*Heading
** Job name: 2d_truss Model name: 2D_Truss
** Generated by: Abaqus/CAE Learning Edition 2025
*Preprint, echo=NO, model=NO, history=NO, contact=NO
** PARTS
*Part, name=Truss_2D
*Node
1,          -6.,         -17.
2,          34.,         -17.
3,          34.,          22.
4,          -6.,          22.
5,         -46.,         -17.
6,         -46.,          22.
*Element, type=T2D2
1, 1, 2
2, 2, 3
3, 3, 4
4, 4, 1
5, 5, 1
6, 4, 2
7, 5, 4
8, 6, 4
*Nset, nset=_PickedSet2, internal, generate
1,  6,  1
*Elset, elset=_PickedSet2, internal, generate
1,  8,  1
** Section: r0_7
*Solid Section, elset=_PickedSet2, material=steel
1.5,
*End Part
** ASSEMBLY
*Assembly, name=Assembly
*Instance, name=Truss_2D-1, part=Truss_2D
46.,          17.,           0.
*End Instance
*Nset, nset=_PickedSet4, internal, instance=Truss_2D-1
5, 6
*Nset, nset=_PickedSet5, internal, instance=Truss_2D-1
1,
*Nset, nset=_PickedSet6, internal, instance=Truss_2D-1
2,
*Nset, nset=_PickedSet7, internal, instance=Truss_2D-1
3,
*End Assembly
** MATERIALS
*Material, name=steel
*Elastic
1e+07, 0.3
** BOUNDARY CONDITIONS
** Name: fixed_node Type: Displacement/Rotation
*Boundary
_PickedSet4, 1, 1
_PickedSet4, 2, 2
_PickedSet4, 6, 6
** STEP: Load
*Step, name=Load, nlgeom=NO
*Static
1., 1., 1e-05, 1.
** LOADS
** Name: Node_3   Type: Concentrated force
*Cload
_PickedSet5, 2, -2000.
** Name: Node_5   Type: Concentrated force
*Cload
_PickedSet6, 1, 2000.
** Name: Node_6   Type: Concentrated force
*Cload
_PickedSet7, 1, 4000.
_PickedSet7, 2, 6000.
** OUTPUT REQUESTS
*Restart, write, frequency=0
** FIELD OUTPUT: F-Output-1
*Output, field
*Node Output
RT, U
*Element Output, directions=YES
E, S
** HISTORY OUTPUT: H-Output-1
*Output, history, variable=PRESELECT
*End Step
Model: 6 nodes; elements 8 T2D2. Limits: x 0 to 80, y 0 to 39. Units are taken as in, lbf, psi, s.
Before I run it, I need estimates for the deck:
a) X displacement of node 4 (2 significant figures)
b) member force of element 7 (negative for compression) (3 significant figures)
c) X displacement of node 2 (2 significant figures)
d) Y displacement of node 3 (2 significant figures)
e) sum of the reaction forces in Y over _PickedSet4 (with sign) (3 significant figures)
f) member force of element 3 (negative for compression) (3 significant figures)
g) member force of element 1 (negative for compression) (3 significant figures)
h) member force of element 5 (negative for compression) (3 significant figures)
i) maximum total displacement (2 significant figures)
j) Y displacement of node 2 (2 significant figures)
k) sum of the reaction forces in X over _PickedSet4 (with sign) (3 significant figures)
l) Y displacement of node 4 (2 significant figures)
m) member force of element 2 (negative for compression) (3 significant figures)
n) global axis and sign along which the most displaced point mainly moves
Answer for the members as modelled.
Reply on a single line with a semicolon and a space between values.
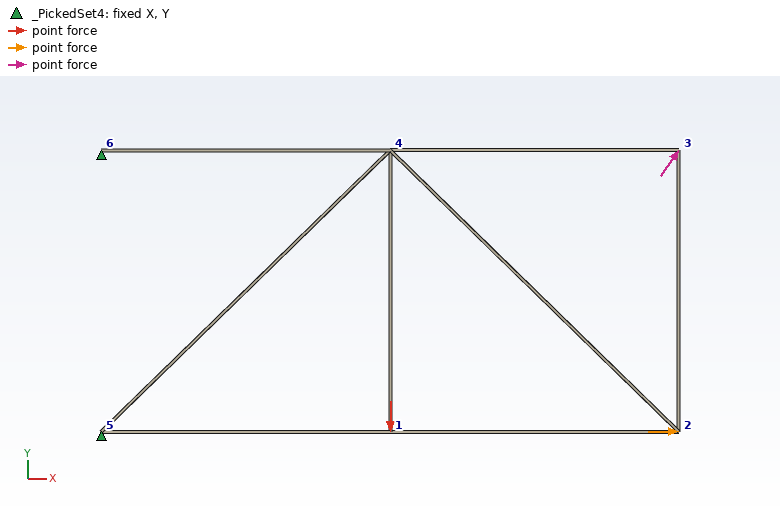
-0.017 in; 5730 lbf; 0.043 in; 0.17 in; -4000 lbf; 4000 lbf; 8150 lbf; 8150 lbf; 0.17 in; 0.16 in; -6000 lbf; 0.048 in; 6000 lbf; +Y
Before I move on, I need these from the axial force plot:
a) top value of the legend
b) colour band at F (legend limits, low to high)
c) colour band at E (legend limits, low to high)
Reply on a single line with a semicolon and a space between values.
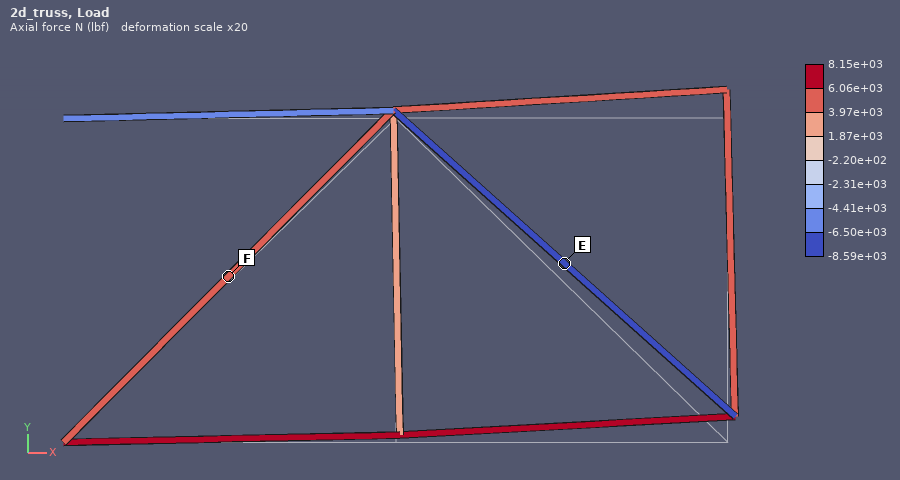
8.15e+03 lbf; 3.97e+03 to 6.06e+03 lbf; -8.59e+03 to -6.50e+03 lbf
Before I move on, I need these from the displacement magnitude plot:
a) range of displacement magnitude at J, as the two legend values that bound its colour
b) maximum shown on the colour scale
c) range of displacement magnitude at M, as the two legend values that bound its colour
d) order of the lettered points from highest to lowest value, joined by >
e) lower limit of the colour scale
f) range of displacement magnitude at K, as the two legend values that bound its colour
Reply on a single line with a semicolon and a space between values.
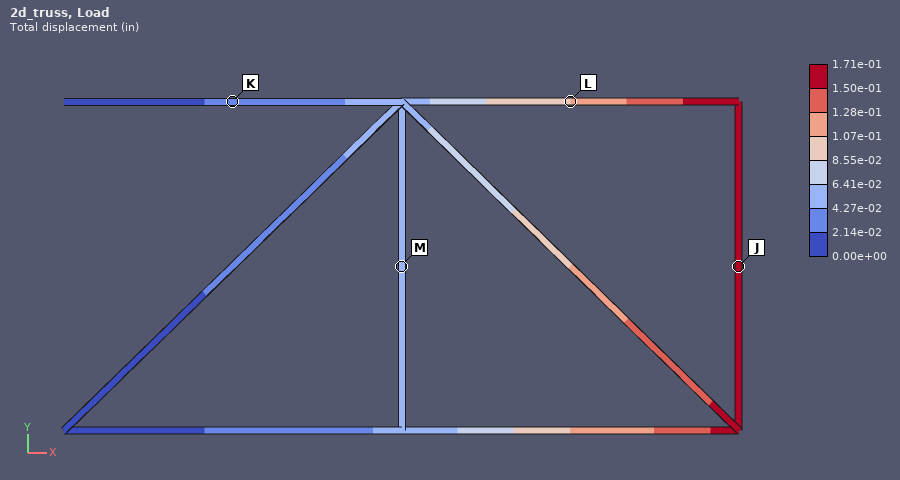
1.50e-01 to 1.71e-01 in; 1.71e-01 in; 4.27e-02 to 6.41e-02 in; J > L > M > K; 0.00e+00 in; 2.14e-02 to 4.27e-02 in
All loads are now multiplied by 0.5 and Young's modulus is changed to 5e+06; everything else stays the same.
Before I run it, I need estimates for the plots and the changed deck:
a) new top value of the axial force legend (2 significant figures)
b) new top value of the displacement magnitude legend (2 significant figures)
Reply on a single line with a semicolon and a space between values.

4100 lbf; 0.17 in
